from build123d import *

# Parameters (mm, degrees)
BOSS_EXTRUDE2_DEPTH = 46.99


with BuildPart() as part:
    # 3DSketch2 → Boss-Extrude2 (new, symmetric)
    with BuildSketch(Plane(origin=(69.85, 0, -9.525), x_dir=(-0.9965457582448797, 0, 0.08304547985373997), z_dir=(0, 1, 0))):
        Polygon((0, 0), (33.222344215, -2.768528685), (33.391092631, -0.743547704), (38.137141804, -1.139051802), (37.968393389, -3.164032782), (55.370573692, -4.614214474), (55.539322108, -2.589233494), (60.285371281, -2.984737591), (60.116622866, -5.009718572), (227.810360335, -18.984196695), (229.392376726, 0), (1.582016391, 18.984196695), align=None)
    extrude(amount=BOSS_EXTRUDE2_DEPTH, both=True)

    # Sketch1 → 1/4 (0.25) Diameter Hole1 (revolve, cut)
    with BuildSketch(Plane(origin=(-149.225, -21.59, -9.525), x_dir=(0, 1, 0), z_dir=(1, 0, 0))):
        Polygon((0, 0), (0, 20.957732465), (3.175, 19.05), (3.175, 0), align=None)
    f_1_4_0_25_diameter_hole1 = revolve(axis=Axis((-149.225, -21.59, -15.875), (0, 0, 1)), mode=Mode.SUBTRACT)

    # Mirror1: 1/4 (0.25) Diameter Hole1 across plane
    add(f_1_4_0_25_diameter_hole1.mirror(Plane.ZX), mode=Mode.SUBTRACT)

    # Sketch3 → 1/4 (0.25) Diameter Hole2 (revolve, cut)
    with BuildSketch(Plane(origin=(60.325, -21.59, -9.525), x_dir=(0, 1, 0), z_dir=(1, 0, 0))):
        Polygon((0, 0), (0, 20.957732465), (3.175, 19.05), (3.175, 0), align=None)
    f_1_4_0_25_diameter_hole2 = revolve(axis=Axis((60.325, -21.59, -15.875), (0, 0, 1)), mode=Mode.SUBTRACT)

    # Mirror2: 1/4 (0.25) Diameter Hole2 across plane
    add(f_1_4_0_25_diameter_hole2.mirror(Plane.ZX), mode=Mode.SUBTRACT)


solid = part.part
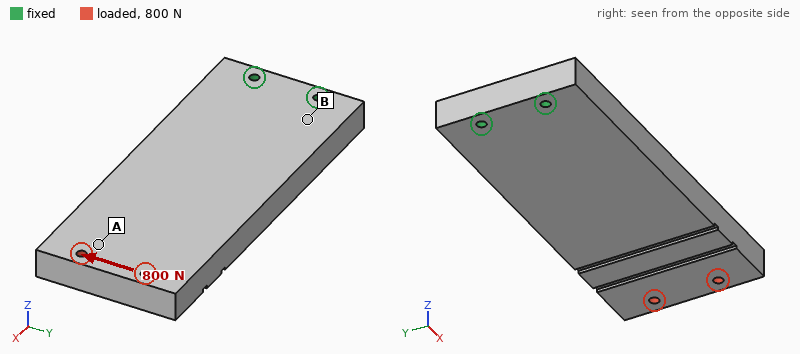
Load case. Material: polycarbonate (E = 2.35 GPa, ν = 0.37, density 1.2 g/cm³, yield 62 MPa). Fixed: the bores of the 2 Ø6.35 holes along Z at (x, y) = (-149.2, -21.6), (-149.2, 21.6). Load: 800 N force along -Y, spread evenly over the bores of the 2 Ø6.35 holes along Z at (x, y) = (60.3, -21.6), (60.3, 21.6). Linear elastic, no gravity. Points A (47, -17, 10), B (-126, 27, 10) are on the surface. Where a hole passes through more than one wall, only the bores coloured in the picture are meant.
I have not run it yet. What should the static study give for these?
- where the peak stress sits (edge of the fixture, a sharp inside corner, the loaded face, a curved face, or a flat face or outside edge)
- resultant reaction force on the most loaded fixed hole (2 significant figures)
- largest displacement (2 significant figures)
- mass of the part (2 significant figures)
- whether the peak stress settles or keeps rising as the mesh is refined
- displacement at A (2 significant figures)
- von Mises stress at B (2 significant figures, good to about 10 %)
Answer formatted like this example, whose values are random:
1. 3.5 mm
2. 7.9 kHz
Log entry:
1. edge of the fixture
2. 3.6 kN
3. 1.6 mm
4. 490 g
5. keeps rising
6. 1.3 mm
7. 5.0 MPa
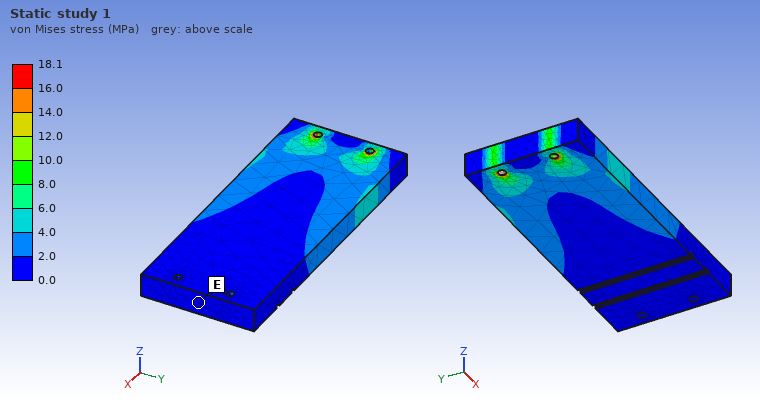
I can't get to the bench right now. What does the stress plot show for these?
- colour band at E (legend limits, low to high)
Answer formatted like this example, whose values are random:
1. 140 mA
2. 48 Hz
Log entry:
1. 0.0 to 2.0 MPa
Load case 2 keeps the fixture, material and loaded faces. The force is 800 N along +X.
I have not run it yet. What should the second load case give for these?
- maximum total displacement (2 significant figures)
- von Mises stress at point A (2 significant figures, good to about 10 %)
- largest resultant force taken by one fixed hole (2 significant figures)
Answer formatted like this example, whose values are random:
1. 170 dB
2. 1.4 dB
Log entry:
1. 54 µm
2. 0.72 MPa
3. 400 N
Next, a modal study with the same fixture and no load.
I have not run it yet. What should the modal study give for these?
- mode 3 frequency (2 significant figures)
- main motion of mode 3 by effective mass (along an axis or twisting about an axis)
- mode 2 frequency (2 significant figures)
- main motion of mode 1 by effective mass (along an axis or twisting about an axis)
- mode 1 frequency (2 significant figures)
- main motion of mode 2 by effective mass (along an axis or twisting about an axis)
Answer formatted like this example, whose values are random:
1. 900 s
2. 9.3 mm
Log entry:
1. 380 Hz
2. twisting about X
3. 300 Hz
4. along Z
5. 85 Hz
6. along Y
